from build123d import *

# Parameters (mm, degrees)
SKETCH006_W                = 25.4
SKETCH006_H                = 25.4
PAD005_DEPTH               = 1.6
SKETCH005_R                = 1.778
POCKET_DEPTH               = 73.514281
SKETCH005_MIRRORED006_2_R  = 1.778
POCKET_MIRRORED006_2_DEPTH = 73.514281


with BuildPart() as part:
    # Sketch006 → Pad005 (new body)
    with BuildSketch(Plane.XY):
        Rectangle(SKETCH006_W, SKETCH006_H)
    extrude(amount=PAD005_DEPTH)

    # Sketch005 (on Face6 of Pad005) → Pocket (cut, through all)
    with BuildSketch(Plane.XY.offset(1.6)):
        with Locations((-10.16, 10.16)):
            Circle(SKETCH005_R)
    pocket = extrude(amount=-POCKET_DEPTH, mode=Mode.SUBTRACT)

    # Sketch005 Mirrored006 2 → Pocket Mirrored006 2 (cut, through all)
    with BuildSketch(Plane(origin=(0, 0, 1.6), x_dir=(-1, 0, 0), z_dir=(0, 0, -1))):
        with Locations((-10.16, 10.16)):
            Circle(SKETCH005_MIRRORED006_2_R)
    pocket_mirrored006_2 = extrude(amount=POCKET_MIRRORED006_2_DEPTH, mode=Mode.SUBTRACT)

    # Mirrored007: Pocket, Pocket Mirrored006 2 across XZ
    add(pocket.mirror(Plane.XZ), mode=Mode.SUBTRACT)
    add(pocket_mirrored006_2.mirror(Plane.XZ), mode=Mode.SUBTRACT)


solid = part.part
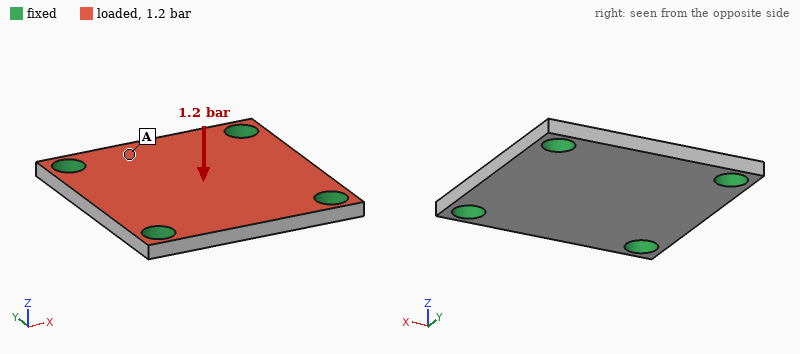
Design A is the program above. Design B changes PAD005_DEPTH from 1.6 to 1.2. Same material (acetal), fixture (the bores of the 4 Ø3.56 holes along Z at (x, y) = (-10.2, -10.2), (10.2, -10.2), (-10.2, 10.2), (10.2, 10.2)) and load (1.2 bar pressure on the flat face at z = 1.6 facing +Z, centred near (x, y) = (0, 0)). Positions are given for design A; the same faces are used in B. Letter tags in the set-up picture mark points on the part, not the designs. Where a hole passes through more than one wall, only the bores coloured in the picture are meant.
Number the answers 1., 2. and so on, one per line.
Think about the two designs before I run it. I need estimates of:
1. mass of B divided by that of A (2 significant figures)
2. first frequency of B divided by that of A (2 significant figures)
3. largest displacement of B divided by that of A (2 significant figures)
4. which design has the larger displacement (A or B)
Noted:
1. 0.75
2. 0.77
3. 2.2
4. B
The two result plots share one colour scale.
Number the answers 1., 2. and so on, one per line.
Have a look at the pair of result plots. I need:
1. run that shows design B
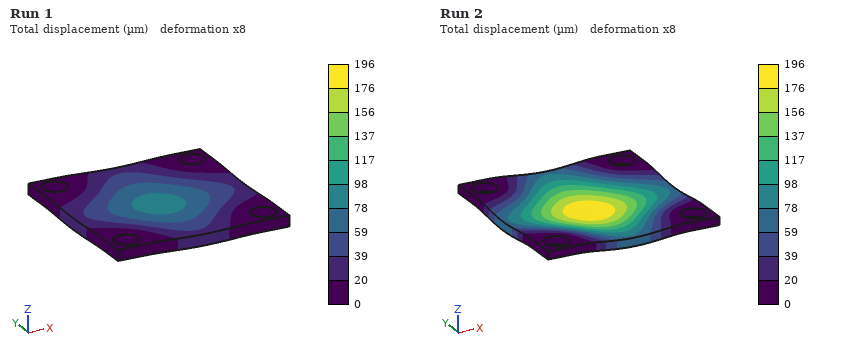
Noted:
1. Run 2
